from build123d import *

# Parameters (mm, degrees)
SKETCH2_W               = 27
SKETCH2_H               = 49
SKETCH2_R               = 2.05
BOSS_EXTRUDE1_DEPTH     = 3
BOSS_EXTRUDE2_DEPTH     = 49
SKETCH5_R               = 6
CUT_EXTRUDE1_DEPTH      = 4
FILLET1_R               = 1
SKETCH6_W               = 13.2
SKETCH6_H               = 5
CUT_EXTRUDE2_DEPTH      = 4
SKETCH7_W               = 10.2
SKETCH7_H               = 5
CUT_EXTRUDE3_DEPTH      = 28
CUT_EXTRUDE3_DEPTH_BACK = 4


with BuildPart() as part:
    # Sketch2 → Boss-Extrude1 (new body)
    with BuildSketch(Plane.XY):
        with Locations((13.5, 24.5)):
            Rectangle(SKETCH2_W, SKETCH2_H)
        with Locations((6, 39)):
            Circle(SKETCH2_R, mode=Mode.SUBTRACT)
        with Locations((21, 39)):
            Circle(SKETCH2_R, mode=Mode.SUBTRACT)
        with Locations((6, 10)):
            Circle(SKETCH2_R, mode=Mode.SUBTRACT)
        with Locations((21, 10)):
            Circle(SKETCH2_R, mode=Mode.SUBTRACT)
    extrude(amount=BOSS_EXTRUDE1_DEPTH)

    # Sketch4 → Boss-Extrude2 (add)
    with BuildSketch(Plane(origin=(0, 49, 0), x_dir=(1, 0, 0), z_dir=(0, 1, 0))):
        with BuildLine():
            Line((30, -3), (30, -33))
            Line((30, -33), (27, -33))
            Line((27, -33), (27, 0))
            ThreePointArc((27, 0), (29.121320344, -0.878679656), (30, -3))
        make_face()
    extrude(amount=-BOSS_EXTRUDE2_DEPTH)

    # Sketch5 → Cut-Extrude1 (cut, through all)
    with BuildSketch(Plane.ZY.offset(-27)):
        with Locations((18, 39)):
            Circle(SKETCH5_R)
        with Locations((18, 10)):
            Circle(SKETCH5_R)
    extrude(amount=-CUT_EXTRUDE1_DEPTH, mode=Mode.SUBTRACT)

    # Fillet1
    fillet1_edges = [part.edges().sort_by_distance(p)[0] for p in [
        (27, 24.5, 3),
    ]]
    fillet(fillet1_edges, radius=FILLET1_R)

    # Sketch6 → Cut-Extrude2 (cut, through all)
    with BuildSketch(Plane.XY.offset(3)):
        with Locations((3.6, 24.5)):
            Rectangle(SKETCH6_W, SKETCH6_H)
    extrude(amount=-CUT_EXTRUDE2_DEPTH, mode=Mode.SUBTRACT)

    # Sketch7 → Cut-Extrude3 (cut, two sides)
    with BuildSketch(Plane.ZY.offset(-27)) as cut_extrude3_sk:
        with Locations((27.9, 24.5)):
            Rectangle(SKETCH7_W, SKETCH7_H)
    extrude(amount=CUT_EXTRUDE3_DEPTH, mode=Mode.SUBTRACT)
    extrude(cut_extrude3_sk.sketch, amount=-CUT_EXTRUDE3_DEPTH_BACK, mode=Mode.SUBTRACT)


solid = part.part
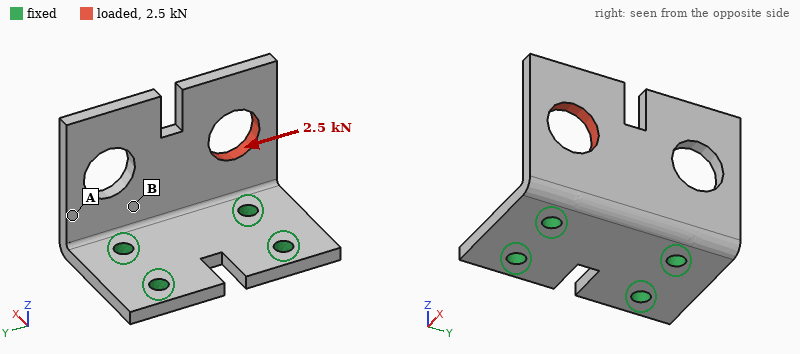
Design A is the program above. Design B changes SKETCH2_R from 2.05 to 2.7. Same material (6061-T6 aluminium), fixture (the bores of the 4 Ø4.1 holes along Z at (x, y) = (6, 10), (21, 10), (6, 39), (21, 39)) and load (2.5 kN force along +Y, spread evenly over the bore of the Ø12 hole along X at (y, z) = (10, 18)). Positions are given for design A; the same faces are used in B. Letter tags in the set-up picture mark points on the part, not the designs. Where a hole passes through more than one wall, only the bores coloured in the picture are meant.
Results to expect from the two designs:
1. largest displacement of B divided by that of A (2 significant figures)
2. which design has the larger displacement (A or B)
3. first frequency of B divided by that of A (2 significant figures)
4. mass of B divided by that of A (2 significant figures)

0.83
A
1.0
0.98
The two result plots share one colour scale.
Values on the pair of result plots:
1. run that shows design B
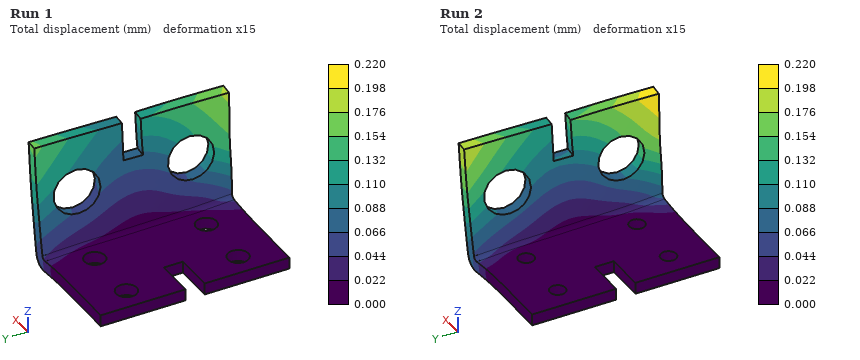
Run 1
